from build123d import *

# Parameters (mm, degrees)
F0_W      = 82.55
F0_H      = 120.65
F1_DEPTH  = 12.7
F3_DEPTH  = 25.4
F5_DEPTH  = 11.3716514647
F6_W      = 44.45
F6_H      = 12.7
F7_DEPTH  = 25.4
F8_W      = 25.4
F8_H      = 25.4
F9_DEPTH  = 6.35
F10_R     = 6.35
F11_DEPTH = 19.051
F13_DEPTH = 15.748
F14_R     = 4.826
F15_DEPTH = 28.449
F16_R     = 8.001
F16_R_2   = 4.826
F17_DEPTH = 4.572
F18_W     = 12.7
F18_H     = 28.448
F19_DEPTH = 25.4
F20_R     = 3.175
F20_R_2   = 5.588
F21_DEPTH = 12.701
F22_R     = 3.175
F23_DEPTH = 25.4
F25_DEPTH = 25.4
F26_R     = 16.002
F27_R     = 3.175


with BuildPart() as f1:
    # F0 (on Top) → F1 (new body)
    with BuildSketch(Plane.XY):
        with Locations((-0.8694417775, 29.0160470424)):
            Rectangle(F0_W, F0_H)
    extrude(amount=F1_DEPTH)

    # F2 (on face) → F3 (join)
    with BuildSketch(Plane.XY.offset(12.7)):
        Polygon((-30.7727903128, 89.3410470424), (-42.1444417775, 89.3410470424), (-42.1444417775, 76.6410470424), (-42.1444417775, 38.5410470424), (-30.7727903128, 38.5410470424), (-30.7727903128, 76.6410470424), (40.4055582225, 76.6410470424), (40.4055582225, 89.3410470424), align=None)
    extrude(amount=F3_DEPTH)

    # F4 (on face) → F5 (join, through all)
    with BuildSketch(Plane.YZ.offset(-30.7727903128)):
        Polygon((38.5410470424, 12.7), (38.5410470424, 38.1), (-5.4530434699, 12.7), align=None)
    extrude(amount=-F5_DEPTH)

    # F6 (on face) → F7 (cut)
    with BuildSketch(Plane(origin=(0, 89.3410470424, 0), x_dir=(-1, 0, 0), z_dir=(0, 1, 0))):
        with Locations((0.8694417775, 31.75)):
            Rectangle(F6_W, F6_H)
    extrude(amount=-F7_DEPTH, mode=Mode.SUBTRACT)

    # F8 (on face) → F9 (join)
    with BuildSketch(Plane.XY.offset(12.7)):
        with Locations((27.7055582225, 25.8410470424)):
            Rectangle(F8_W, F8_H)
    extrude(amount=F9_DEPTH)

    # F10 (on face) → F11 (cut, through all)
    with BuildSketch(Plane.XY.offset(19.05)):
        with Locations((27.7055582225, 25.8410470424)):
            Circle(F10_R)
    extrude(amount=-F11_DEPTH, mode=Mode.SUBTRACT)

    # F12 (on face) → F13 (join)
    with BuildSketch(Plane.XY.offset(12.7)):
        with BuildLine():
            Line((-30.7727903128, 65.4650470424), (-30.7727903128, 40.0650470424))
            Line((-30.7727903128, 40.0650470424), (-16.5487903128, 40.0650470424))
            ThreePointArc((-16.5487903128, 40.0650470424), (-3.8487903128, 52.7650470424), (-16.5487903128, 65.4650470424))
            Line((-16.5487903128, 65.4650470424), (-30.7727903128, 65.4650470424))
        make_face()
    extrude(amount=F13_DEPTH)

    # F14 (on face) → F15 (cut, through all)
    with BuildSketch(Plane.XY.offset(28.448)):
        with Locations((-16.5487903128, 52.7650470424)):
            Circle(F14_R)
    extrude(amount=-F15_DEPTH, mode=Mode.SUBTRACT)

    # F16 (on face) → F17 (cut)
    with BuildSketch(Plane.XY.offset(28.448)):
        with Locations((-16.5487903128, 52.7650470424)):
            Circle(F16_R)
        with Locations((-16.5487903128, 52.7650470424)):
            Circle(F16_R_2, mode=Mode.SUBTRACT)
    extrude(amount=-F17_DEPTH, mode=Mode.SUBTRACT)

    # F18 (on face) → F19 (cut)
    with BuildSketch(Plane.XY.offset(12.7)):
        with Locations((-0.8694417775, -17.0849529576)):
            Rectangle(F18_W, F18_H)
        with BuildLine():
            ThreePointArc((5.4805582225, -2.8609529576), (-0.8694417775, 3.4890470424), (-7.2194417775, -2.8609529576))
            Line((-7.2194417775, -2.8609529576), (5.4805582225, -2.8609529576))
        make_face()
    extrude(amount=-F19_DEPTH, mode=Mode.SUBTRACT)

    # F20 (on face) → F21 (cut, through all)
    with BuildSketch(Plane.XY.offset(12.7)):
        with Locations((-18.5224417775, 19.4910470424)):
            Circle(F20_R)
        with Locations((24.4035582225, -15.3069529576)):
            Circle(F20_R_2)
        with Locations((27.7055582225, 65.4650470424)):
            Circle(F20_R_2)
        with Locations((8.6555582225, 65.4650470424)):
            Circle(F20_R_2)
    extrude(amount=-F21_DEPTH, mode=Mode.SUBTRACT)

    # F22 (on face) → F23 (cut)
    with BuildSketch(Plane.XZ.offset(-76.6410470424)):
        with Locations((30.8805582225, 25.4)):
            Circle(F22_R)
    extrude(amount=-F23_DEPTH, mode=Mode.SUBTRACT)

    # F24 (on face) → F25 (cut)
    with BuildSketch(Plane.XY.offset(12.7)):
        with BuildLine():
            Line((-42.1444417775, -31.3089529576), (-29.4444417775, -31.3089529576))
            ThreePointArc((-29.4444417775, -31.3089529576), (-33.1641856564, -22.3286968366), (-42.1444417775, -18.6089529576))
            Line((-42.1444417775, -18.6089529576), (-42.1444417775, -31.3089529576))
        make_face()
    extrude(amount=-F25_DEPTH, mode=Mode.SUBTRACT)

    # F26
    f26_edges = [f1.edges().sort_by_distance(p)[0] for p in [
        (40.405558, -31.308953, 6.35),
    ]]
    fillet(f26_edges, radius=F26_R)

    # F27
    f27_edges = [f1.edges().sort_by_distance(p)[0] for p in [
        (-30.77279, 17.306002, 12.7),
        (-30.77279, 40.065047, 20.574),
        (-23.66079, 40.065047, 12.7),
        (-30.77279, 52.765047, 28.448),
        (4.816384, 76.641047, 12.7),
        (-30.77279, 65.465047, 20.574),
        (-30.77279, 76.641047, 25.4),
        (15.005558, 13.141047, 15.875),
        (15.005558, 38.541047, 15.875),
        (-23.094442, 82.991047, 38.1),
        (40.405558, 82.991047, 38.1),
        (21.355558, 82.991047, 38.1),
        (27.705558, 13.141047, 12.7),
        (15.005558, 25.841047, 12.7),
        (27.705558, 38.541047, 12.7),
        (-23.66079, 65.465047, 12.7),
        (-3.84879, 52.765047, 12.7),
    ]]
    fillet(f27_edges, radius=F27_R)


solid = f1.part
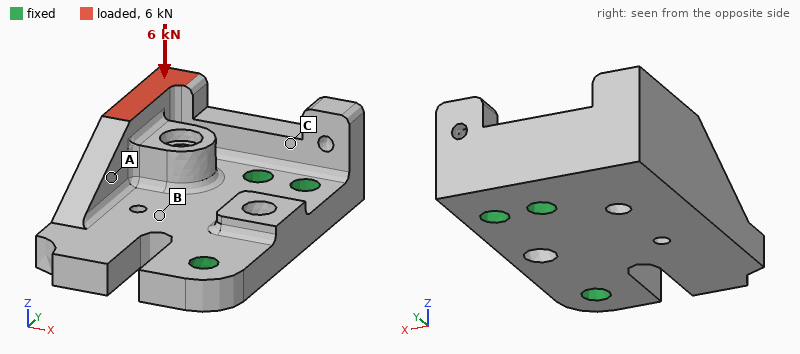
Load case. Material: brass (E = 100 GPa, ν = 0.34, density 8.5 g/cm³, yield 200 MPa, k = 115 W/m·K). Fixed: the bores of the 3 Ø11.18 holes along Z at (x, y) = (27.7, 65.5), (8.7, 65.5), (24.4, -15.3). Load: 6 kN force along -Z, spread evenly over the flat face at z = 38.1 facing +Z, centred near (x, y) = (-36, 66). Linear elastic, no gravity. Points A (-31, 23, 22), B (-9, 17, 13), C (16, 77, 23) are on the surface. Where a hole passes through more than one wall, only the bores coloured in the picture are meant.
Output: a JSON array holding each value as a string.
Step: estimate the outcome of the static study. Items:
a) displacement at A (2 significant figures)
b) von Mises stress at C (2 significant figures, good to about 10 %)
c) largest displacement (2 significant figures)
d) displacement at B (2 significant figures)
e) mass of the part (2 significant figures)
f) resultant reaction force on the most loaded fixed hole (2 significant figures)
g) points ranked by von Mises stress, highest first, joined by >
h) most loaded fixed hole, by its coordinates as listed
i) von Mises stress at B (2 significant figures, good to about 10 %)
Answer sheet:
["0.087 mm", "36 MPa", "0.14 mm", "0.035 mm", "1.4 kg", "11 kN", "C > B > A", "(8.7, 65.5)", "23 MPa"]
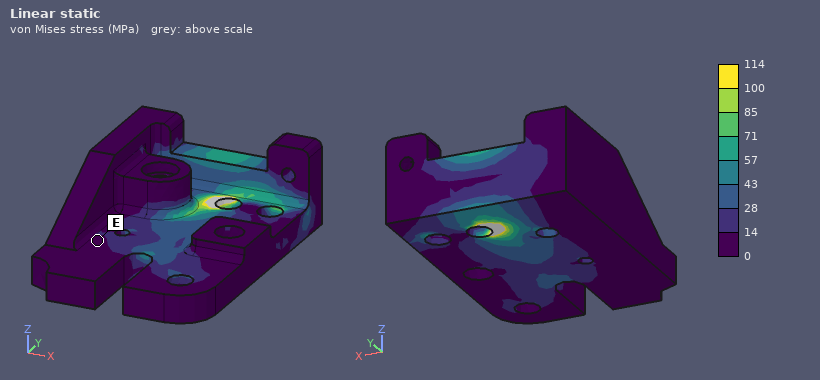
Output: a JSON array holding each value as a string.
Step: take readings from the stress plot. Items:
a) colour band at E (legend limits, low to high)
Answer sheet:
["0 to 14 MPa"]
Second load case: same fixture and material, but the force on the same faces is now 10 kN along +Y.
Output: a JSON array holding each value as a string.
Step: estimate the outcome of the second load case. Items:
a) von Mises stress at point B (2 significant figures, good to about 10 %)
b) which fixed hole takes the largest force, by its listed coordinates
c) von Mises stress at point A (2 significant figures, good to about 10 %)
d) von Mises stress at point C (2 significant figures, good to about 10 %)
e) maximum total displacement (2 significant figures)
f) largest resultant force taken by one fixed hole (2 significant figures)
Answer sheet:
["63 MPa", "(8.7, 65.5)", "46 MPa", "29 MPa", "0.22 mm", "11 kN"]
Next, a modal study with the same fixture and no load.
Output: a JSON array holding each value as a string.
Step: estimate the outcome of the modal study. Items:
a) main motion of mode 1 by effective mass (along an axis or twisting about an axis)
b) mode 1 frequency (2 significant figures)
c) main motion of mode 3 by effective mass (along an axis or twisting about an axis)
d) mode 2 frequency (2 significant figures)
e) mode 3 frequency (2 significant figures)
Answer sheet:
["along Z", "1400 Hz", "along Y", "2300 Hz", "3600 Hz"]
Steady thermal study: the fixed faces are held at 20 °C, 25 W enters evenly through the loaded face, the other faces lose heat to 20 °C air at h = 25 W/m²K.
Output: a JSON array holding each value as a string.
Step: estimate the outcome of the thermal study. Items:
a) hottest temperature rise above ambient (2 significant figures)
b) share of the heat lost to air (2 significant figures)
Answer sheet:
["14 K", "12 %"]
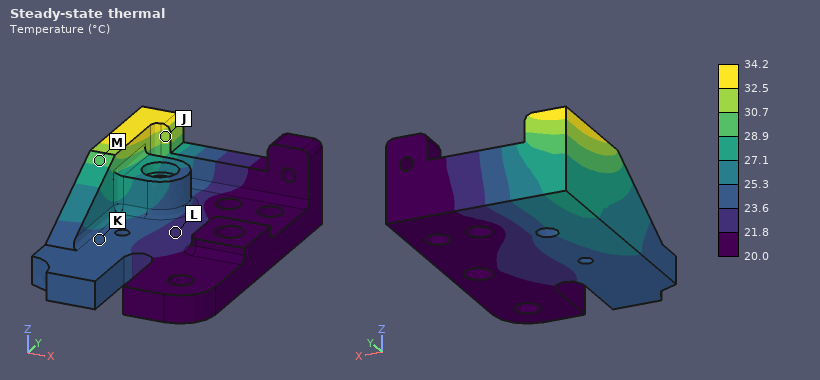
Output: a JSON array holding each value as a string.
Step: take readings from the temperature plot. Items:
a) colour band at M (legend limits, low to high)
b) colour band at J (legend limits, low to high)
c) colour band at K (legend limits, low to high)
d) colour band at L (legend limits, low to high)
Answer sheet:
["28.9 to 30.7 °C", "30.7 to 32.5 °C", "23.6 to 25.3 °C", "21.8 to 23.6 °C"]
